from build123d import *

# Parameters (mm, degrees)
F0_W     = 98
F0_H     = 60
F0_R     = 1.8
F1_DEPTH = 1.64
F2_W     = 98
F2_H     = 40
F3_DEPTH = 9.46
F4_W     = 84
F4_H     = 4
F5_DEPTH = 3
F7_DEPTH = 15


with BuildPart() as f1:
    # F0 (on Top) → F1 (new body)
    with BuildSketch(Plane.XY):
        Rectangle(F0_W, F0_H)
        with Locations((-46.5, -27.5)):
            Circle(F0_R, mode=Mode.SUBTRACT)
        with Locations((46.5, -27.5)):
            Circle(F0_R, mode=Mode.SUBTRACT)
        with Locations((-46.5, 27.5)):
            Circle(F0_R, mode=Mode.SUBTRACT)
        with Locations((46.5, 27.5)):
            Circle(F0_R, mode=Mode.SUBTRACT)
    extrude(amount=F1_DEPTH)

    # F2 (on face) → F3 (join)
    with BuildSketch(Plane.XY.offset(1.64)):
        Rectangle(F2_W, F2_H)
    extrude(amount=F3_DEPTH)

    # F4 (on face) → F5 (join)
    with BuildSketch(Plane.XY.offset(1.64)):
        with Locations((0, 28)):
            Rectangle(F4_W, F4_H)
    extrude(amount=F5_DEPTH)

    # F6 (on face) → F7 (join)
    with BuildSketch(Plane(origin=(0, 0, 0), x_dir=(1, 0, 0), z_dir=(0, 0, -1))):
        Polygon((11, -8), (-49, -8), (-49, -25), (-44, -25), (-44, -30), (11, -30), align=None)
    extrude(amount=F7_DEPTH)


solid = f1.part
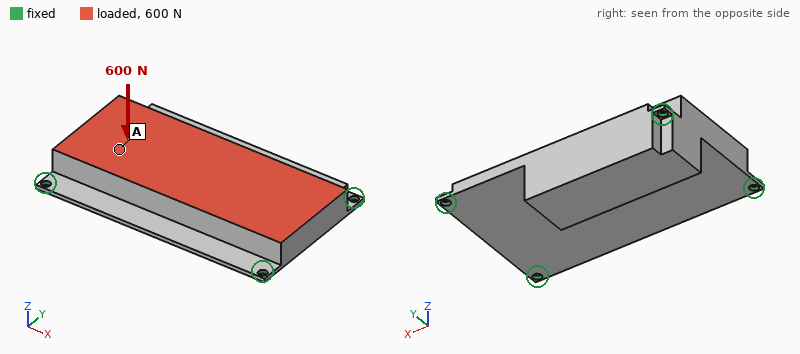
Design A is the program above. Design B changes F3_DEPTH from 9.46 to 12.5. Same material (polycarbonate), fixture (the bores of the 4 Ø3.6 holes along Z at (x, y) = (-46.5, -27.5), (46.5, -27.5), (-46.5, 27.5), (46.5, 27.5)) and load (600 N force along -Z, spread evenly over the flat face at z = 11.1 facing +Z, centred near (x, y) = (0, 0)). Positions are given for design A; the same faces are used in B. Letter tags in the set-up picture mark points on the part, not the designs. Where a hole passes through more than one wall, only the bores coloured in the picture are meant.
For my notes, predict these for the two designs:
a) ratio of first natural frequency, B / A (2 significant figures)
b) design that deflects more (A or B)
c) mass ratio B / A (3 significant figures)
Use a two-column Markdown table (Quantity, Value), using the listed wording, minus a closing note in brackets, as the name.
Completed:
| Quantity | Value |
|---|---|
| ratio of first natural frequency, B / A | 0.98 |
| design that deflects more | A |
| mass ratio B / A | 1.18 |
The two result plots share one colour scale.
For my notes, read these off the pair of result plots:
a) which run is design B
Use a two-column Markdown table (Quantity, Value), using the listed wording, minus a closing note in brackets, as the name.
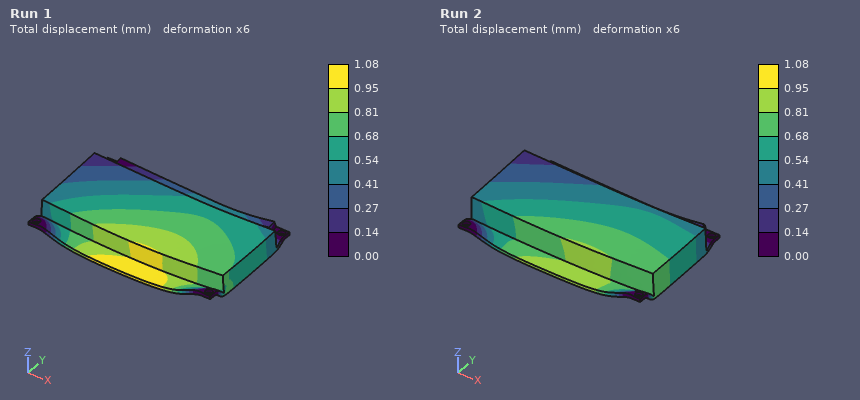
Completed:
| Quantity | Value |
|---|---|
| which run is design B | Run 2 |
